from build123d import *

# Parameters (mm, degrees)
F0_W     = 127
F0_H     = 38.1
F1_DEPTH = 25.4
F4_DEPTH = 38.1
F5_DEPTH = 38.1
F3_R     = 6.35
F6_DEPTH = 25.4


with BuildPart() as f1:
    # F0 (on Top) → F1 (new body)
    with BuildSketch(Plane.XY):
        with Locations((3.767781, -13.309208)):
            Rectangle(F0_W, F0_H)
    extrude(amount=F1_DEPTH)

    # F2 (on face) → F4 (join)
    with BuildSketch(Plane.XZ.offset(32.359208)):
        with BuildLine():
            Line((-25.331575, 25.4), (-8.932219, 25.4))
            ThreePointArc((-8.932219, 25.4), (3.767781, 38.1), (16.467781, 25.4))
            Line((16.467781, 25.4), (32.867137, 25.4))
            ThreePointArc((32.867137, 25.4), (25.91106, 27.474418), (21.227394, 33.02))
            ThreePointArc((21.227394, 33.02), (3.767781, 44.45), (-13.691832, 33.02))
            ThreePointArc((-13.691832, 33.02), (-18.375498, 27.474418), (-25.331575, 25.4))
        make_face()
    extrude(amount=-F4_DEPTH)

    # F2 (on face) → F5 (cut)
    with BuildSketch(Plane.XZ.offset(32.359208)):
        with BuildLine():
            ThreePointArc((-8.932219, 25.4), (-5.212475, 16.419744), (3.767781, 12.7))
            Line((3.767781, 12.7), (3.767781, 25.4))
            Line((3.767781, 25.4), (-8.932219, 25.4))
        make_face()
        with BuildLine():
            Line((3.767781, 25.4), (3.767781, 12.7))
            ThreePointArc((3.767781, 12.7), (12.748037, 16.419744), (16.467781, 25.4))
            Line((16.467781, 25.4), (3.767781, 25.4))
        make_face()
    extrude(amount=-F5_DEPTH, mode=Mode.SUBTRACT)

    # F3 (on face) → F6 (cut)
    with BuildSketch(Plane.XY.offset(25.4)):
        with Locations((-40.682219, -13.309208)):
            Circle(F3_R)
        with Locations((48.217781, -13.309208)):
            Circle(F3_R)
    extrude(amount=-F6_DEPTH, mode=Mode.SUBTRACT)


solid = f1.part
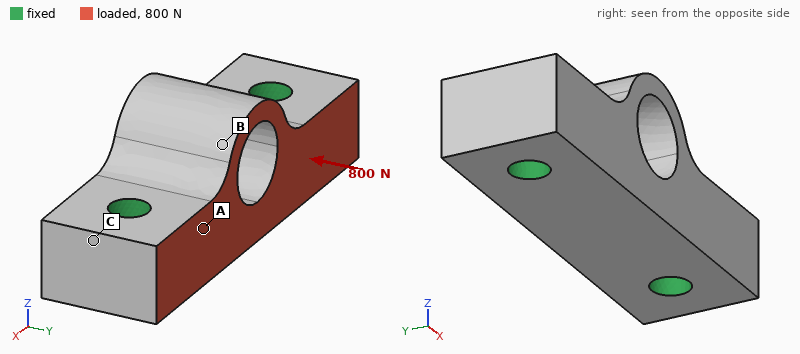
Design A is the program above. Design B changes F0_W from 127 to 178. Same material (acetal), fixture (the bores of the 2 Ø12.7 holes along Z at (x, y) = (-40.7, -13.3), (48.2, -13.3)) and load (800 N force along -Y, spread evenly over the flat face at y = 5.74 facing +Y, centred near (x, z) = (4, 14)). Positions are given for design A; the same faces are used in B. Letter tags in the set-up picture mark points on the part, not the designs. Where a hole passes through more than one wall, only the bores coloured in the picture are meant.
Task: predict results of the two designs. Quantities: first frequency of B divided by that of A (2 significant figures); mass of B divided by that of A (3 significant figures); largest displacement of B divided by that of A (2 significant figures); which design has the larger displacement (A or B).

0.80
1.41
0.66
A
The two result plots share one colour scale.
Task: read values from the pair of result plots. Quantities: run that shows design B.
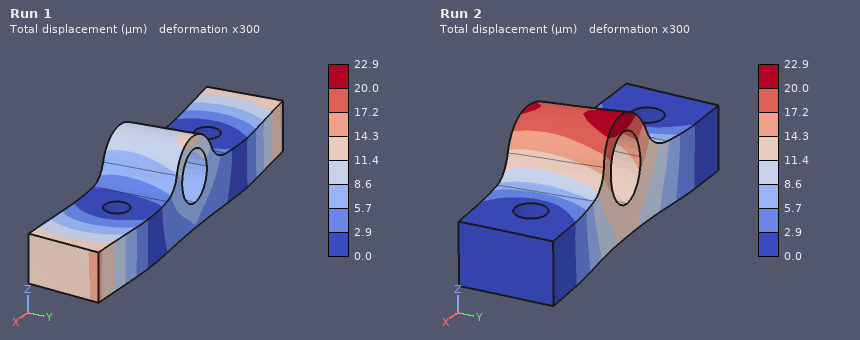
Run 1
